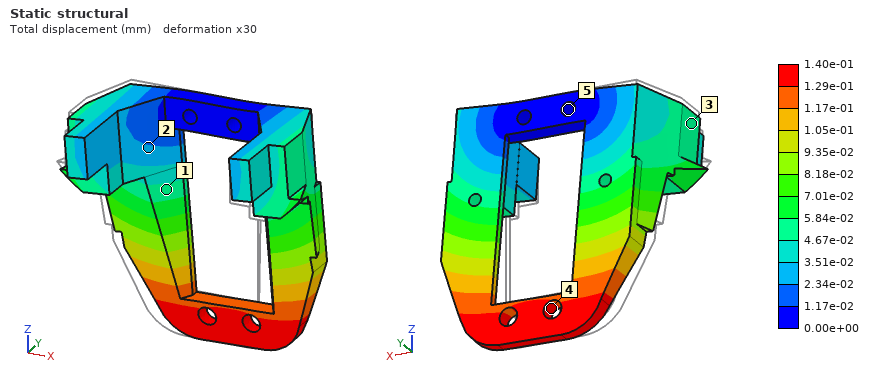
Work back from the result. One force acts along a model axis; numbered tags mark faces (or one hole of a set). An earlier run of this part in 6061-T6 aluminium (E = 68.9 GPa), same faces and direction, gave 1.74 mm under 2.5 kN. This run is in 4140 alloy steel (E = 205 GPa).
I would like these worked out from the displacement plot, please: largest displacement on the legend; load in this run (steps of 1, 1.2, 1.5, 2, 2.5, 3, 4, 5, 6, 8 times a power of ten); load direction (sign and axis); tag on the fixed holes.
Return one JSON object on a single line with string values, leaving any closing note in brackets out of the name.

{"largest displacement on the legend": "1.40e-01 mm", "load in this run": "600 N", "load direction": "+X", "tag on the fixed holes": "5"}
